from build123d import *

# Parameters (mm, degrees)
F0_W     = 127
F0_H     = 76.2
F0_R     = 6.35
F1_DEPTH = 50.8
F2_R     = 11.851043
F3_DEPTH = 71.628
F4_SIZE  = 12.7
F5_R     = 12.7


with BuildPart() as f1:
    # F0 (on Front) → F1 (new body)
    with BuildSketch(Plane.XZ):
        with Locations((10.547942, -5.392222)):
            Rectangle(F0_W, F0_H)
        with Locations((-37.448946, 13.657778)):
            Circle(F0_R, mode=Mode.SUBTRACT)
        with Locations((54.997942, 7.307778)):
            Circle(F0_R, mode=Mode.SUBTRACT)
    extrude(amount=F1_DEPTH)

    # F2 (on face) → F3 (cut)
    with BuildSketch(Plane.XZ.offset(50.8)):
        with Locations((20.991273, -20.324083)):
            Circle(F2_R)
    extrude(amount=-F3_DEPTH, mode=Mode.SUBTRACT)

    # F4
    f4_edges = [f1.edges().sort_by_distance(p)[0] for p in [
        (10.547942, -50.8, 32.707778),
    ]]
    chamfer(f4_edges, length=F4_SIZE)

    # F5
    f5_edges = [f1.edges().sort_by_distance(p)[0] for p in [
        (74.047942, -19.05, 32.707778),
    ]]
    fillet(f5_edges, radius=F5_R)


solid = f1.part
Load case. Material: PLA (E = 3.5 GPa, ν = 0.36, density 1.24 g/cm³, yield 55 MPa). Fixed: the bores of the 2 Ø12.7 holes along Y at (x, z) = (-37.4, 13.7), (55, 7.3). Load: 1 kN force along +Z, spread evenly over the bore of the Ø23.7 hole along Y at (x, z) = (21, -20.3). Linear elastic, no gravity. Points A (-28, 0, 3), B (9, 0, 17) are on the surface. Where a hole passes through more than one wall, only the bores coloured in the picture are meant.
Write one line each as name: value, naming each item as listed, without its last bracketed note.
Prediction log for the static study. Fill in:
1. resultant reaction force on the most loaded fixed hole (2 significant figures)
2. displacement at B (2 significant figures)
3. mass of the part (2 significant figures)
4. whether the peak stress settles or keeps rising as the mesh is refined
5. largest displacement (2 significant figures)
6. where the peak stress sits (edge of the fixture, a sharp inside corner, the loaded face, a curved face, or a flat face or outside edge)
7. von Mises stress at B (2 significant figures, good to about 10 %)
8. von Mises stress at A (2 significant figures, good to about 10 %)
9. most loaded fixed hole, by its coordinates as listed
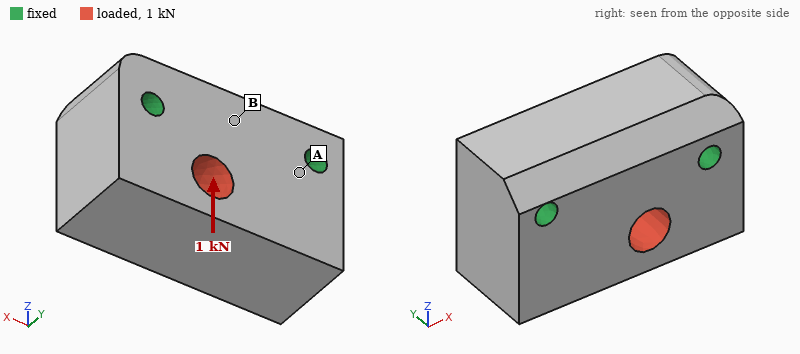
resultant reaction force on the most loaded fixed hole: 650 N
displacement at B: 5.4 µm
mass of the part: 550 g
whether the peak stress settles or keeps rising as the mesh is refined: keeps rising
largest displacement: 9.1 µm
where the peak stress sits: edge of the fixture
von Mises stress at B: 0.12 MPa
von Mises stress at A: 0.34 MPa
most loaded fixed hole, by its coordinates as listed: (55, 7.3)
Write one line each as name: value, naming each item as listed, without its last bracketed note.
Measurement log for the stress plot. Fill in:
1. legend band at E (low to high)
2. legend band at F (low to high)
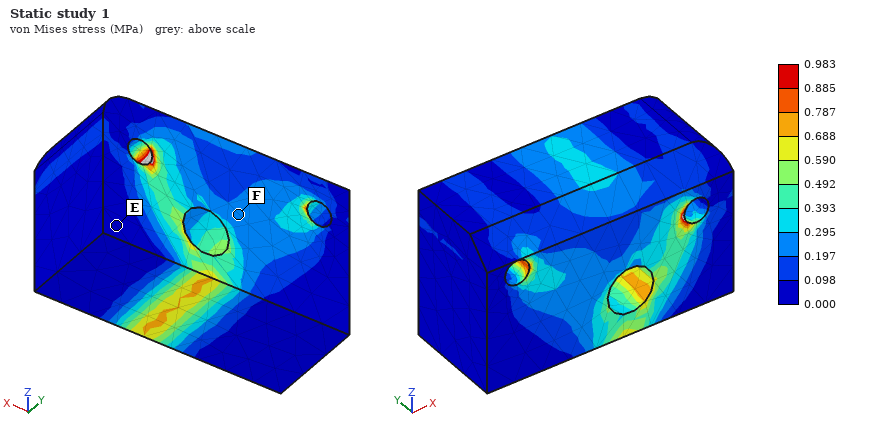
legend band at E: 0.000 to 0.098 MPa
legend band at F: 0.197 to 0.295 MPa
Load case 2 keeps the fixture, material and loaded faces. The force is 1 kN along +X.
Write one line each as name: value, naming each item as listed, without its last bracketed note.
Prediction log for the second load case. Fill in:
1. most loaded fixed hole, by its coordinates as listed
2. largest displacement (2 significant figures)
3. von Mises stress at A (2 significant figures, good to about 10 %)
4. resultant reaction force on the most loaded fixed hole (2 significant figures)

most loaded fixed hole, by its coordinates as listed: (55, 7.3)
largest displacement: 8.7 µm
von Mises stress at A: 0.32 MPa
resultant reaction force on the most loaded fixed hole: 650 N
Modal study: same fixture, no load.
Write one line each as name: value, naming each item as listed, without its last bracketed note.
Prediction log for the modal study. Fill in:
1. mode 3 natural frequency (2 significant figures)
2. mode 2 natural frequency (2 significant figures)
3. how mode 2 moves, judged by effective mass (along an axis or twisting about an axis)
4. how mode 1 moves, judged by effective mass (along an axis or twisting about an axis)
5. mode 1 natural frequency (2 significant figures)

mode 3 natural frequency: 3700 Hz
mode 2 natural frequency: 3400 Hz
how mode 2 moves, judged by effective mass: along X
how mode 1 moves, judged by effective mass: along Y
mode 1 natural frequency: 2500 Hz
